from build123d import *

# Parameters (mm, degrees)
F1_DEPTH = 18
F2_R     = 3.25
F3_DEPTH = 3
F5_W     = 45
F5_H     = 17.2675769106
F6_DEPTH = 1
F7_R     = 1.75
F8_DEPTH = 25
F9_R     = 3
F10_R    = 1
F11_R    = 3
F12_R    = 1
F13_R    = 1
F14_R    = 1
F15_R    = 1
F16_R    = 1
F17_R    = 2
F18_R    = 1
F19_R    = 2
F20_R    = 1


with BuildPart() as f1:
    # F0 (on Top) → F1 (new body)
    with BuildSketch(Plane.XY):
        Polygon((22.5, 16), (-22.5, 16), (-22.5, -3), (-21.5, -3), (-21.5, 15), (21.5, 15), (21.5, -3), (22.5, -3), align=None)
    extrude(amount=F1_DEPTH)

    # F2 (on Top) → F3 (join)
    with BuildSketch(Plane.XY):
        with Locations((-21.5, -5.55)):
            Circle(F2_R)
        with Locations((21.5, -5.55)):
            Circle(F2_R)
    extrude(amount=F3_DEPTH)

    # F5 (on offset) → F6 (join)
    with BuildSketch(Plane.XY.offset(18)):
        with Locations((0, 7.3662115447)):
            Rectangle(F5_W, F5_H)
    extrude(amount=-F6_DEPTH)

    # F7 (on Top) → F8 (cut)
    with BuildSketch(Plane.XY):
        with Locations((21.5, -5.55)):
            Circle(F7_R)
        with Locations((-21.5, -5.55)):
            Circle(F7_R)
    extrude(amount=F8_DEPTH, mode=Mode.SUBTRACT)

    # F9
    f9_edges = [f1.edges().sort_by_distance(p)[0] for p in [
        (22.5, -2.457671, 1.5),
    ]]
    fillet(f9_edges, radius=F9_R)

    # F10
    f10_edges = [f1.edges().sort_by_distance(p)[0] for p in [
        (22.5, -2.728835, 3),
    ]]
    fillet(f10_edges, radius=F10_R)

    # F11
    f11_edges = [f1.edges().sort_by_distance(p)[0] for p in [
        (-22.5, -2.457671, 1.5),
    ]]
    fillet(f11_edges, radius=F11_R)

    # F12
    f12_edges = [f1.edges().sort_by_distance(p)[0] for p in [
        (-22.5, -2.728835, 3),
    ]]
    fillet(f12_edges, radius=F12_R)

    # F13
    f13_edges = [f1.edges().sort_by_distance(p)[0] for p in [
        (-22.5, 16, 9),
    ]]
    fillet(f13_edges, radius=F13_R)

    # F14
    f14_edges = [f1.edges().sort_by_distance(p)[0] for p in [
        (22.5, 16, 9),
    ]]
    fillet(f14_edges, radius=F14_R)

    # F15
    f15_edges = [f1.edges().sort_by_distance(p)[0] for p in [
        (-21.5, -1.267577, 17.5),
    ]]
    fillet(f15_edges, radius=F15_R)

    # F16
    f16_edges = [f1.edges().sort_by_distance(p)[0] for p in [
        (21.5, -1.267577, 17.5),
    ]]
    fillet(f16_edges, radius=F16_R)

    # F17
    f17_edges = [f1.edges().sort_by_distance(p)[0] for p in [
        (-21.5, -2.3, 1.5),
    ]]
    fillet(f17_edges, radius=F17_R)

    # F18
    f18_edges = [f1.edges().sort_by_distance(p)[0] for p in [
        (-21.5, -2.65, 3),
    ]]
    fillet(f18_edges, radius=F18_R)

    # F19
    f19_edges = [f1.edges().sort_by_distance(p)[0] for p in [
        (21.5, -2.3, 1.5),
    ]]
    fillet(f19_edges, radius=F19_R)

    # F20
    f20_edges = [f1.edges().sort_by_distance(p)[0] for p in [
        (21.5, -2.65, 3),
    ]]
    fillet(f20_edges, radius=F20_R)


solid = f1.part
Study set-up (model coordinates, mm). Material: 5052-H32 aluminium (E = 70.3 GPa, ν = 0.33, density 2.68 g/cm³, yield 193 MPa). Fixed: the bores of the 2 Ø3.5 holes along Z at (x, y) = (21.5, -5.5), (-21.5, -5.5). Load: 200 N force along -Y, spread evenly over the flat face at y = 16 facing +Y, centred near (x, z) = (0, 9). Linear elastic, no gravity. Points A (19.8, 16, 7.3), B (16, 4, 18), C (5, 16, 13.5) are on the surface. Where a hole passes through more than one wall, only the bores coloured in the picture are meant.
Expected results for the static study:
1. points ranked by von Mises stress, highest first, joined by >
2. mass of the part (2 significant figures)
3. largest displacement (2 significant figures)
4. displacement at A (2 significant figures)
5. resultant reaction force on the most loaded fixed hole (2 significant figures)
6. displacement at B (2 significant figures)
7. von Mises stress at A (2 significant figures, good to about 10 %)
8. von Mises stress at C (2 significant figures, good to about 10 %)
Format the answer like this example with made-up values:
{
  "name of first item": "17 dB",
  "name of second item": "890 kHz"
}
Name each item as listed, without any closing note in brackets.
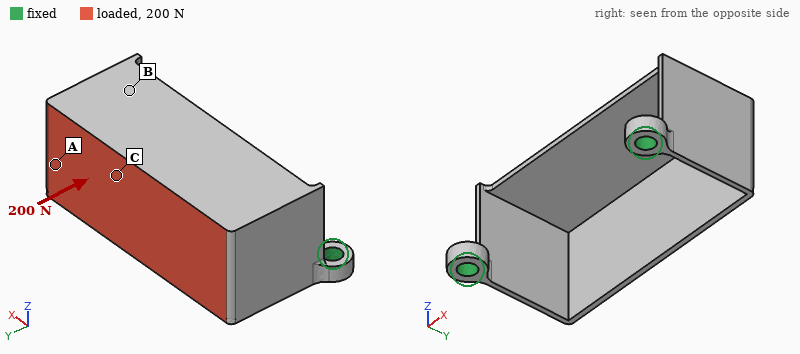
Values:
{
  "points ranked by von Mises stress, highest first, joined by >": "A > C > B",
  "mass of the part": "6.1 g",
  "largest displacement": "0.37 mm",
  "displacement at A": "0.15 mm",
  "resultant reaction force on the most loaded fixed hole": "100 N",
  "displacement at B": "0.14 mm",
  "von Mises stress at A": "70 MPa",
  "von Mises stress at C": "39 MPa"
}
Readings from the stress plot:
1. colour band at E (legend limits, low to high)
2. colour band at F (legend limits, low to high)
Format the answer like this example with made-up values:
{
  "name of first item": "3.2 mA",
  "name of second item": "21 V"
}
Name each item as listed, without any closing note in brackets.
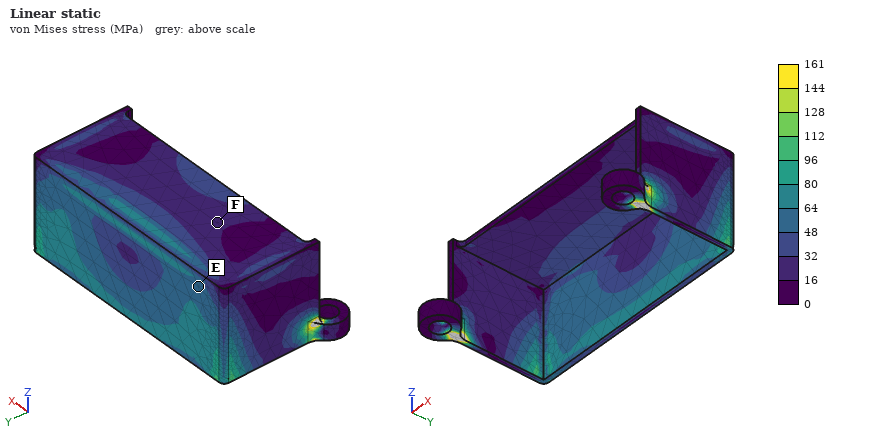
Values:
{
  "colour band at E": "48 to 64 MPa",
  "colour band at F": "16 to 32 MPa"
}
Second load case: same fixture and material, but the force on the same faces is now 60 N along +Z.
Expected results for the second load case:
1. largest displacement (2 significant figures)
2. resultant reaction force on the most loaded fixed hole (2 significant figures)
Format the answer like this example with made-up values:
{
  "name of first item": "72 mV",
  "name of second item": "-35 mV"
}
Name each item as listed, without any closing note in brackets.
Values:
{
  "largest displacement": "0.14 mm",
  "resultant reaction force on the most loaded fixed hole": "30 N"
}
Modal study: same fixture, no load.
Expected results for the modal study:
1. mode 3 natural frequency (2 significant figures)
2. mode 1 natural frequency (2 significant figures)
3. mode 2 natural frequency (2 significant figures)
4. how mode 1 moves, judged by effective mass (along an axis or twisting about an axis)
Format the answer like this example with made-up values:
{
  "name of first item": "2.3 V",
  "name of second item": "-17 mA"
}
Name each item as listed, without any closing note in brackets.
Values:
{
  "mode 3 natural frequency": "2500 Hz",
  "mode 1 natural frequency": "1300 Hz",
  "mode 2 natural frequency": "1600 Hz",
  "how mode 1 moves, judged by effective mass": "along X"
}
